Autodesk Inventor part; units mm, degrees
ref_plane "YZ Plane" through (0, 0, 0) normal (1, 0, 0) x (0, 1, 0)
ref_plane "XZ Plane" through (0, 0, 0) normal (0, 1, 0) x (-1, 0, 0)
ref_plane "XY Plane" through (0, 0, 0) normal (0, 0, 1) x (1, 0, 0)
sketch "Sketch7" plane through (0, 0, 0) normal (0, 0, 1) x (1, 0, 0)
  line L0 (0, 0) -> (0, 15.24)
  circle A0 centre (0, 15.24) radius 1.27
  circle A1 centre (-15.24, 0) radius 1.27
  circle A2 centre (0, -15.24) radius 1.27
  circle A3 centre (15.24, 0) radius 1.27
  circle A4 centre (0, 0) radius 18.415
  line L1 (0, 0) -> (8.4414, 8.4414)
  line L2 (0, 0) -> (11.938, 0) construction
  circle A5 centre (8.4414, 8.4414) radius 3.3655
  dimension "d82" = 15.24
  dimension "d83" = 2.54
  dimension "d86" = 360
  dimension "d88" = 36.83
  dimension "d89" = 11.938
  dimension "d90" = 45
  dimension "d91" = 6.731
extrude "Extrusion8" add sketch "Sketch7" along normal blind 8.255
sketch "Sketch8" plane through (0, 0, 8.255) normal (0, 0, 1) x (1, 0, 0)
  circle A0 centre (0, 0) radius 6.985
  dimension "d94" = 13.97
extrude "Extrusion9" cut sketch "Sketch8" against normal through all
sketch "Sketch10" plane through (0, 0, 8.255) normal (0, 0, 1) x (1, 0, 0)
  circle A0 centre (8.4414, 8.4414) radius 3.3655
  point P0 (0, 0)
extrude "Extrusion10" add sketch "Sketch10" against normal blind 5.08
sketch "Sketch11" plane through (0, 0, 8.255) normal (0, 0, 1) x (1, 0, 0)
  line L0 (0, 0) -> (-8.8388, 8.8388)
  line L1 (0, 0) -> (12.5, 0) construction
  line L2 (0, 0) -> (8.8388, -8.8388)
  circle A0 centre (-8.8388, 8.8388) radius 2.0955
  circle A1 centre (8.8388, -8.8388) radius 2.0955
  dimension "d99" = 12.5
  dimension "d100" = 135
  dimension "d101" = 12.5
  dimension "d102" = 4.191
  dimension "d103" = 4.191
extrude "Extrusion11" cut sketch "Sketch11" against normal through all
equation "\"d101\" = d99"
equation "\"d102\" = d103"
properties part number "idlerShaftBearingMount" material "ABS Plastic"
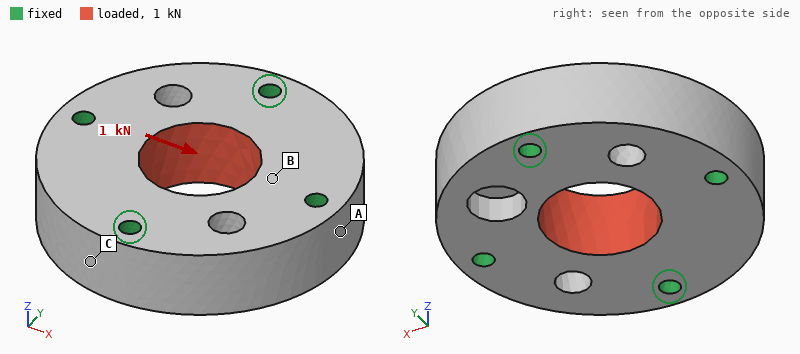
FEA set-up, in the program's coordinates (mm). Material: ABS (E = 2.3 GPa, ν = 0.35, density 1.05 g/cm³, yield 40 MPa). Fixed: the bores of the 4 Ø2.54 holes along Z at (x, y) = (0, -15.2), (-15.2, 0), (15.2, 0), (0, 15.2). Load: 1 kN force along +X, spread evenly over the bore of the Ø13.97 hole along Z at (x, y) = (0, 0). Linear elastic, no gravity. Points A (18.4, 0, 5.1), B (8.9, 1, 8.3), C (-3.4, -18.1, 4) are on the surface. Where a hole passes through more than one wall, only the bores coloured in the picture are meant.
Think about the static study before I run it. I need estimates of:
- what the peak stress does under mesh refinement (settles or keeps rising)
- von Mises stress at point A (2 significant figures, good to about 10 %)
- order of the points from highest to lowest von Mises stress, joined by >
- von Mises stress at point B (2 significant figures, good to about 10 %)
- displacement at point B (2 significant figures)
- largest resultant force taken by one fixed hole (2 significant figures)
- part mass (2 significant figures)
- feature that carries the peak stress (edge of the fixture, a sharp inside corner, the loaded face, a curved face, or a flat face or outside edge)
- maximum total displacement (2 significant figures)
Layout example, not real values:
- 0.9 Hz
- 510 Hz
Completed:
- keeps rising
- 2.8 MPa
- B > A > C
- 4.4 MPa
- 12 µm
- 300 N
- 7.4 g
- edge of the fixture
- 31 µm
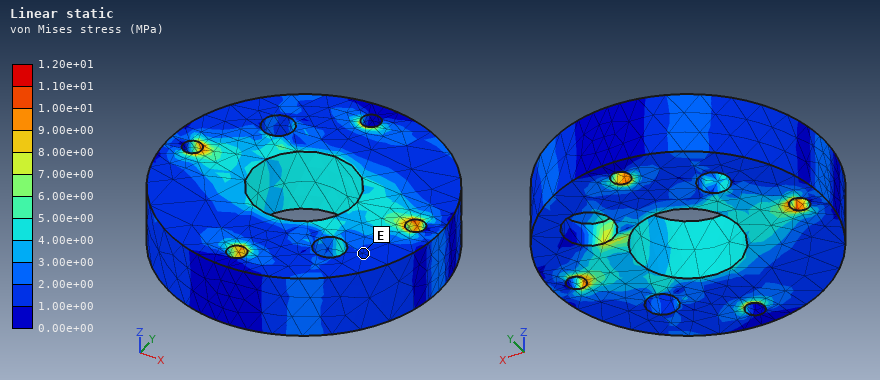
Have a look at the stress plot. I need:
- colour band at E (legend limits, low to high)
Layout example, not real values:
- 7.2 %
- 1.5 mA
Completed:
- 1.00e+00 to 2.00e+00 MPa
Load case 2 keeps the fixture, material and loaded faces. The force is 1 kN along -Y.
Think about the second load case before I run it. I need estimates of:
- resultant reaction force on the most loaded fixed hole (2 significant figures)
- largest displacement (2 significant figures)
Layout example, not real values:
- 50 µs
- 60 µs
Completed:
- 300 N
- 31 µm
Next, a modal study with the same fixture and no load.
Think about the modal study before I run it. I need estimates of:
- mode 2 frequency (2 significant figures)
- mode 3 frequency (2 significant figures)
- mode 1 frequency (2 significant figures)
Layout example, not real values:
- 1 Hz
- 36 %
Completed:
- 14 kHz
- 14 kHz
- 13 kHz
